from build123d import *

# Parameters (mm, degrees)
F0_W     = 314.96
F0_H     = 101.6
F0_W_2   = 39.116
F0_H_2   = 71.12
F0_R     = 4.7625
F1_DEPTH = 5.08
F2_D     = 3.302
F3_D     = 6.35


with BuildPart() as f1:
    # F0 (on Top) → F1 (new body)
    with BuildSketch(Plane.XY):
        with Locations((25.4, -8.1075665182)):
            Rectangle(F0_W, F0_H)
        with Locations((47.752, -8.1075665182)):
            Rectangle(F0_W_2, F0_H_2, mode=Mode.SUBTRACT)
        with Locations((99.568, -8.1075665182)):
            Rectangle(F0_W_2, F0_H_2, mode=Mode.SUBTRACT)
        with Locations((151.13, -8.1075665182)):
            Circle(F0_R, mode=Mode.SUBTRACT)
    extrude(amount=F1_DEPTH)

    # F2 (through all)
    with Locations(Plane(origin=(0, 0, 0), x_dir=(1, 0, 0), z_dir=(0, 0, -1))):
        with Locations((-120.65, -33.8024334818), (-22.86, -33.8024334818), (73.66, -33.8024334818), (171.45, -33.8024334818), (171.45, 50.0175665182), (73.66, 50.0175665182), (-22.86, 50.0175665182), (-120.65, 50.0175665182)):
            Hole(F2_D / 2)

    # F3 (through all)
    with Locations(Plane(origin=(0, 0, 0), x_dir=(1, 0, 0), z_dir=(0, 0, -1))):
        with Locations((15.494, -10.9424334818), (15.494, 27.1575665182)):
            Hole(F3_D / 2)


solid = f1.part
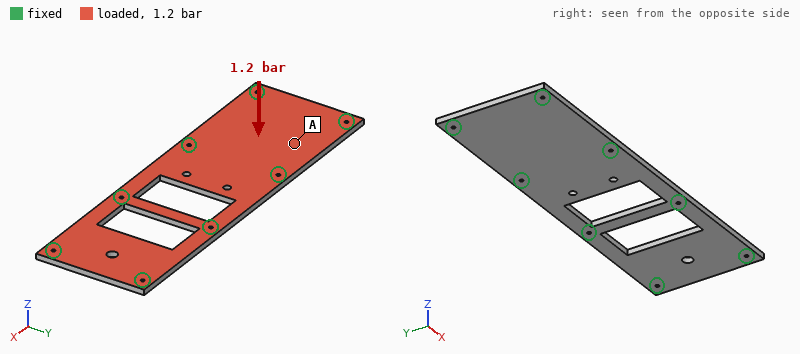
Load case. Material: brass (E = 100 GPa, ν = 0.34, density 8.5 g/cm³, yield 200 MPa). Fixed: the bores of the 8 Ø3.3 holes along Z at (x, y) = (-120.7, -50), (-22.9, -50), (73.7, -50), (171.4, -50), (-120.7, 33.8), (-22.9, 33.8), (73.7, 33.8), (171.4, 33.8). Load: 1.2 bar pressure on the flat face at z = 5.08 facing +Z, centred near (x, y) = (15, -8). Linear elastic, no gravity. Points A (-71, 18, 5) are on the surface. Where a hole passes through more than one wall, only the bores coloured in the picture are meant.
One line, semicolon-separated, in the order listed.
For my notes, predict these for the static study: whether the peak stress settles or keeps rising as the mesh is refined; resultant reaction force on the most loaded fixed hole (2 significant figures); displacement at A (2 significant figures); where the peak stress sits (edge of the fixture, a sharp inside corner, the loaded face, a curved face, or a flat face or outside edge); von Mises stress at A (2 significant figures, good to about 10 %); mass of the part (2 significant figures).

keeps rising; 590 N; 46 µm; edge of the fixture; 12 MPa; 1.1 kg
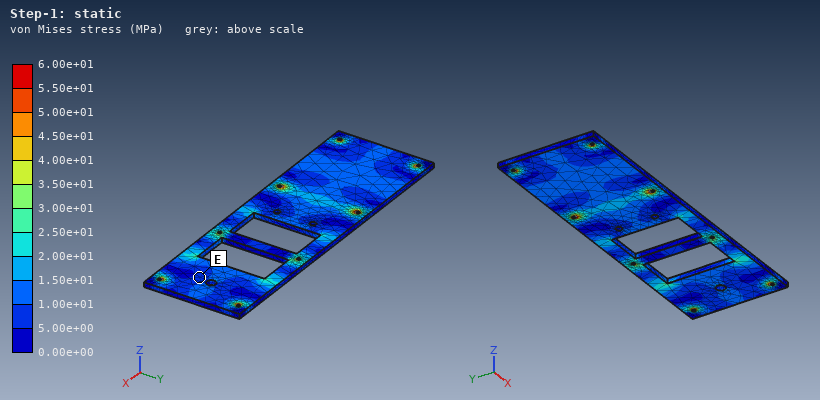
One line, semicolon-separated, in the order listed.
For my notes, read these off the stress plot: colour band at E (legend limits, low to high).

5.00e+00 to 1.00e+01 MPa
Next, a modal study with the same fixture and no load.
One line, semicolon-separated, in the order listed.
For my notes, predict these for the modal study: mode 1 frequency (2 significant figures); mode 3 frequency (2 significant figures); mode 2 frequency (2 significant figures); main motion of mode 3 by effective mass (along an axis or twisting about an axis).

1200 Hz; 1300 Hz; 1200 Hz; along Z
